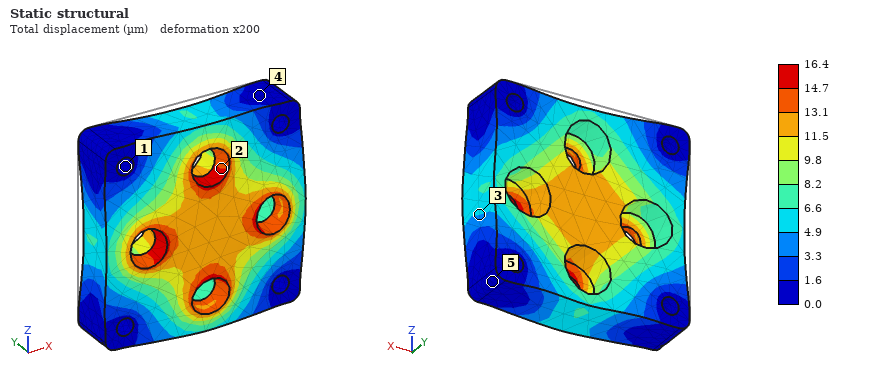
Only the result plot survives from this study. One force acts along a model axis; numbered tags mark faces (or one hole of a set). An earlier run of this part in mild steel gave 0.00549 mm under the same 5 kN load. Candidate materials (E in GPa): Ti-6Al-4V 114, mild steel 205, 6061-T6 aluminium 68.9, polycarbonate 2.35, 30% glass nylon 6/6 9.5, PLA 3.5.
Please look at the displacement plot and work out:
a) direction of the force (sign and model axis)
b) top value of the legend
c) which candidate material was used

-Y
16.4 µm
6061-T6 aluminium
